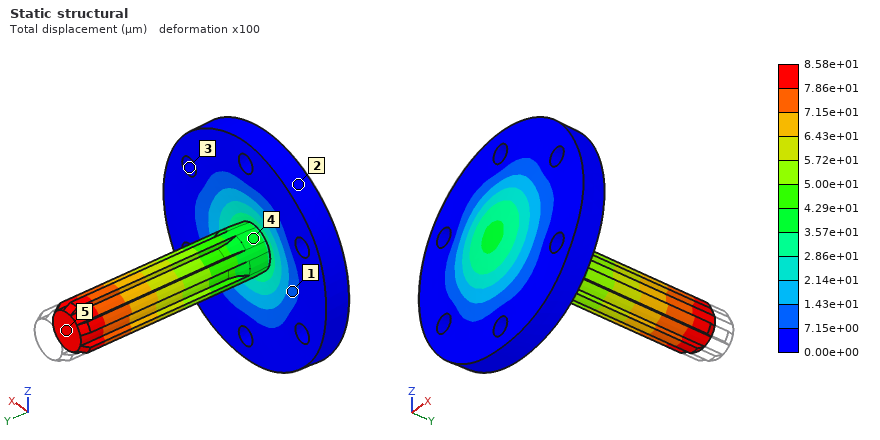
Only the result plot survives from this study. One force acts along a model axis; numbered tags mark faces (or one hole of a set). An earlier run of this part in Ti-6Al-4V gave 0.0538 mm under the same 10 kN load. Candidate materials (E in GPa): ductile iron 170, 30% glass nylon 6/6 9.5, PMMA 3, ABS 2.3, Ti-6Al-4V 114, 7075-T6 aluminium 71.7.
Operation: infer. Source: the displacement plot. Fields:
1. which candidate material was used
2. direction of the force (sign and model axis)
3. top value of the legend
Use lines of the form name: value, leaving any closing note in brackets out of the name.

which candidate material was used: 7075-T6 aluminium
direction of the force: -Y
top value of the legend: 8.58e+01 µm
